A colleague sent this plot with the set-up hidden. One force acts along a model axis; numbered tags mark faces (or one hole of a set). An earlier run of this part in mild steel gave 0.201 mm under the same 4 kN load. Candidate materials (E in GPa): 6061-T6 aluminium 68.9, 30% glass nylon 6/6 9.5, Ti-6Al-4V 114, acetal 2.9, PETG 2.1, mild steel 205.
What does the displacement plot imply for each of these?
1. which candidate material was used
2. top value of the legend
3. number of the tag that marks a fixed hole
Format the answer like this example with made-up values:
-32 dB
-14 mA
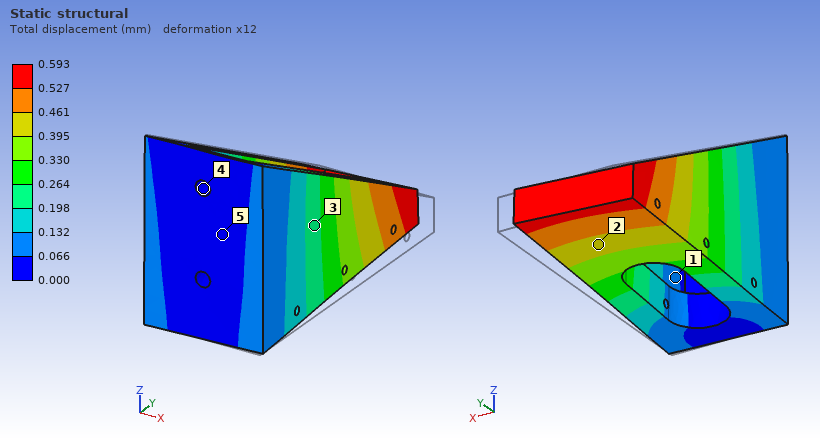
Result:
6061-T6 aluminium
0.593 mm
4
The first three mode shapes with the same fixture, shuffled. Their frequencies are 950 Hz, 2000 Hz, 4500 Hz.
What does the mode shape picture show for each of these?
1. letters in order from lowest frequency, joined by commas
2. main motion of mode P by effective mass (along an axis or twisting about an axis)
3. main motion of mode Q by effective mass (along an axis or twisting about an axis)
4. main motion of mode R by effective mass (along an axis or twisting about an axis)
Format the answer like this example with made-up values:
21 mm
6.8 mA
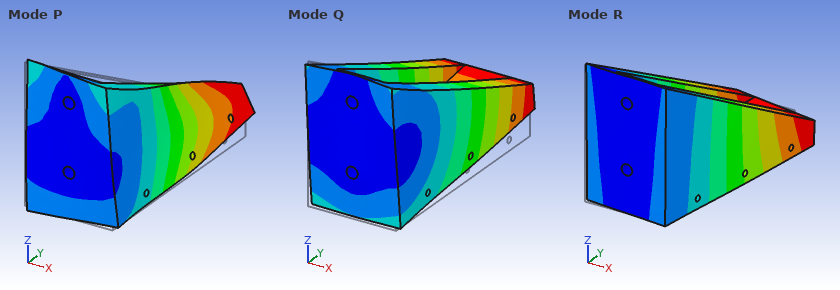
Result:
R, Q, P
twisting about Y
along Z
along X
